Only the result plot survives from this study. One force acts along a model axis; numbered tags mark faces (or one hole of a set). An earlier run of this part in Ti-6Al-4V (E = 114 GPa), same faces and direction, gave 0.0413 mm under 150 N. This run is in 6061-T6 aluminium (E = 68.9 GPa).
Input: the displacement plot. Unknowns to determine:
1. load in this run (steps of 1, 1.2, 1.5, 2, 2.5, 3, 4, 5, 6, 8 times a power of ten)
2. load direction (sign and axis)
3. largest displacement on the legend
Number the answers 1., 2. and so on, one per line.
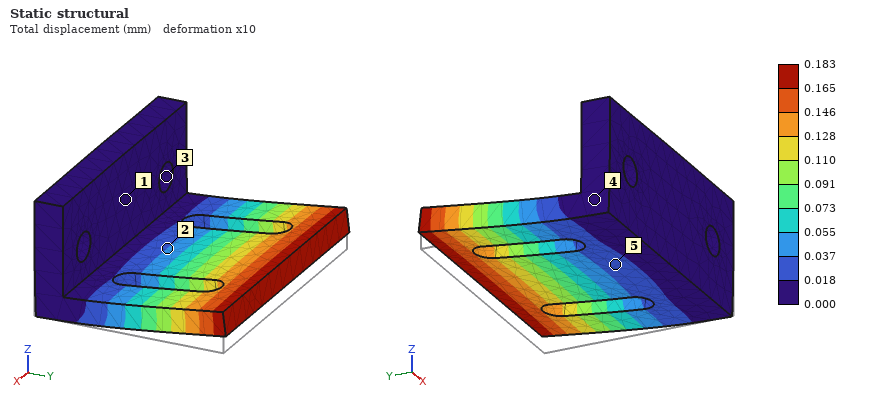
1. 400 N
2. +Z
3. 0.183 mm
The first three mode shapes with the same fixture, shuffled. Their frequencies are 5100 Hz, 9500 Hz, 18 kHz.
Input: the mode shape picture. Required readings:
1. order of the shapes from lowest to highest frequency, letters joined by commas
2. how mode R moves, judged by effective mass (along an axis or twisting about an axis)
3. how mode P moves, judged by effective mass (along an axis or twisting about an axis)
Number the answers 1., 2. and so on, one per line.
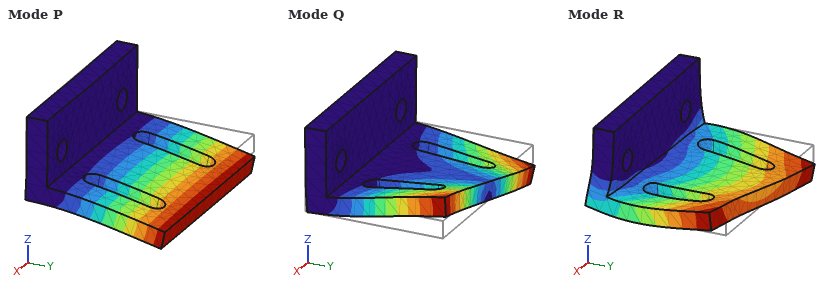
1. P, Q, R
2. along X
3. along Z
